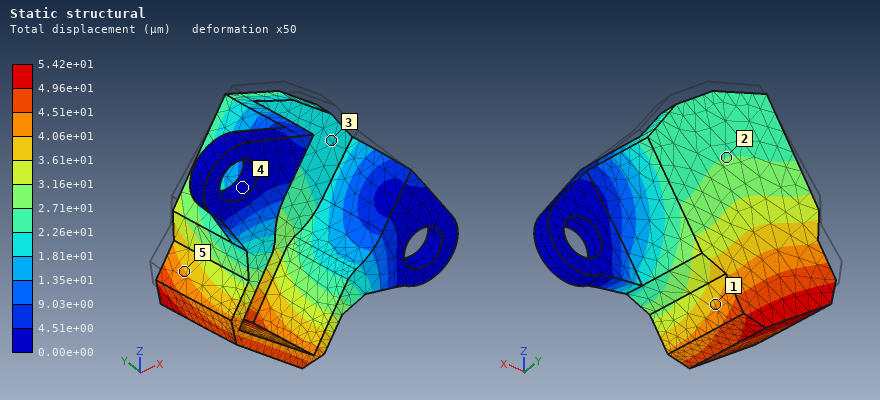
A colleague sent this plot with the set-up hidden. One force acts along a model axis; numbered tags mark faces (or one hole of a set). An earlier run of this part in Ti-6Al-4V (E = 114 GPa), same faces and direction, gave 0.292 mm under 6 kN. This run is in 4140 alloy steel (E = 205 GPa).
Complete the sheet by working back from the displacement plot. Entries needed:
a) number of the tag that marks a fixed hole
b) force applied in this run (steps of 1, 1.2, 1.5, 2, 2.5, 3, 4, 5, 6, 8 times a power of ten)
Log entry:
4
2 kN
